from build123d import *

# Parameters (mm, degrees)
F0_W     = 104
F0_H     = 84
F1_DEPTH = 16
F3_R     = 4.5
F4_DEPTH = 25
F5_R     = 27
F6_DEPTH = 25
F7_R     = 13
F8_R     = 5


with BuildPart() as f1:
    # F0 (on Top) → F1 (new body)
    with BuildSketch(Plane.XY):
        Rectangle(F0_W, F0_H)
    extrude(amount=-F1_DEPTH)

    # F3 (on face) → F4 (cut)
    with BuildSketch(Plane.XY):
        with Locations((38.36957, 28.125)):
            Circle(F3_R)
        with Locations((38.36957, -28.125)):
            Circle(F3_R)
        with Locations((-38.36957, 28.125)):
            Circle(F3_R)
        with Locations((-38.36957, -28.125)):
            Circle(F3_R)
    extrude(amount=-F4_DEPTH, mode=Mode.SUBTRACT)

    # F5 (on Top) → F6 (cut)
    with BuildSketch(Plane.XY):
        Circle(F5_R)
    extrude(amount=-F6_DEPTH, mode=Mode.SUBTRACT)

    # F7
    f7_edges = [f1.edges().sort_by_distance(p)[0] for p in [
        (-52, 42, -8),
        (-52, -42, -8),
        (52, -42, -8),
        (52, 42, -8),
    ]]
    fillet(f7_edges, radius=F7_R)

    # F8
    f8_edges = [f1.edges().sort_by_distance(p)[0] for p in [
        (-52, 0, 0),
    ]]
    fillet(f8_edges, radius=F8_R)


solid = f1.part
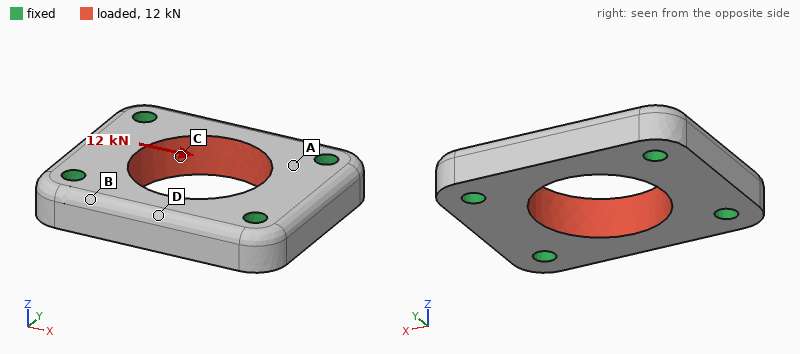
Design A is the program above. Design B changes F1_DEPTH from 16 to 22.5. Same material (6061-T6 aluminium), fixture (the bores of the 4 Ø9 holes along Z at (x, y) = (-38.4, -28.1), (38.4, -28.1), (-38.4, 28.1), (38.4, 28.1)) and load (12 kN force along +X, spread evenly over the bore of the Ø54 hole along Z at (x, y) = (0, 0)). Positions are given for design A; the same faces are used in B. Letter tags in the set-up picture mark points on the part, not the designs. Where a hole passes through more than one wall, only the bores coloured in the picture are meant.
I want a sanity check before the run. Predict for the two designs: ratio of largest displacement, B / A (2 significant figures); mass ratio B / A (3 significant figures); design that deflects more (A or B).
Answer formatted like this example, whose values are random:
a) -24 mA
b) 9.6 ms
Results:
a) 0.72
b) 1.41
c) A
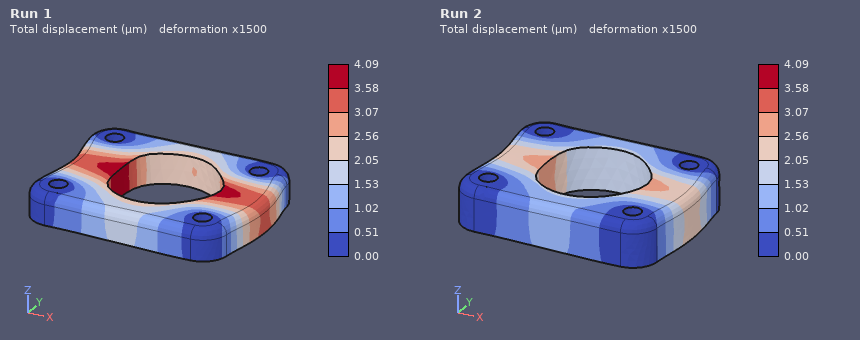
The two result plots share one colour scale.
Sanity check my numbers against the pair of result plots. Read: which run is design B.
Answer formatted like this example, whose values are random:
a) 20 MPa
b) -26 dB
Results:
a) Run 2
